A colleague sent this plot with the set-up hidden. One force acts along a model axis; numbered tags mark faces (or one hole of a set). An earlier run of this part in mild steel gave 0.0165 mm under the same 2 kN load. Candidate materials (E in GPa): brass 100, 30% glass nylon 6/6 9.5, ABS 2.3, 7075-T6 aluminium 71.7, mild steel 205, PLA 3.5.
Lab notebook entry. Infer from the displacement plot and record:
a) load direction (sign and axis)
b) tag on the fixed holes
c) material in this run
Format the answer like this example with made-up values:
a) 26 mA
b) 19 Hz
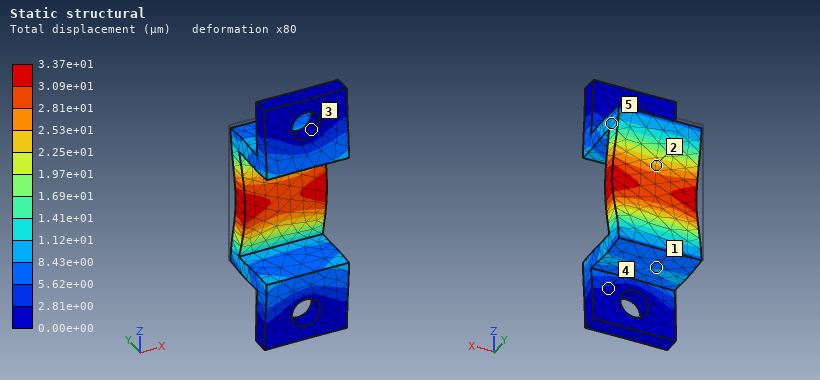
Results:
a) -Y
b) 3
c) brass
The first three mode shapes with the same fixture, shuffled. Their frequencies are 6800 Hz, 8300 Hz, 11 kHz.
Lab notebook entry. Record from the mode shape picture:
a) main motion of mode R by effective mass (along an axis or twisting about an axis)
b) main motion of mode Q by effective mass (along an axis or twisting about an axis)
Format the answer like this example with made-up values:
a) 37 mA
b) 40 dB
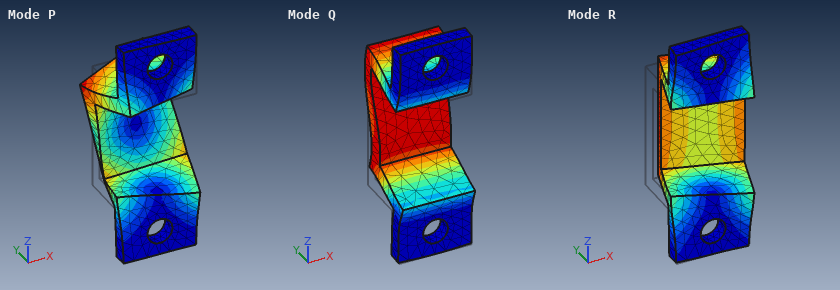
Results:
a) along X
b) along Z
